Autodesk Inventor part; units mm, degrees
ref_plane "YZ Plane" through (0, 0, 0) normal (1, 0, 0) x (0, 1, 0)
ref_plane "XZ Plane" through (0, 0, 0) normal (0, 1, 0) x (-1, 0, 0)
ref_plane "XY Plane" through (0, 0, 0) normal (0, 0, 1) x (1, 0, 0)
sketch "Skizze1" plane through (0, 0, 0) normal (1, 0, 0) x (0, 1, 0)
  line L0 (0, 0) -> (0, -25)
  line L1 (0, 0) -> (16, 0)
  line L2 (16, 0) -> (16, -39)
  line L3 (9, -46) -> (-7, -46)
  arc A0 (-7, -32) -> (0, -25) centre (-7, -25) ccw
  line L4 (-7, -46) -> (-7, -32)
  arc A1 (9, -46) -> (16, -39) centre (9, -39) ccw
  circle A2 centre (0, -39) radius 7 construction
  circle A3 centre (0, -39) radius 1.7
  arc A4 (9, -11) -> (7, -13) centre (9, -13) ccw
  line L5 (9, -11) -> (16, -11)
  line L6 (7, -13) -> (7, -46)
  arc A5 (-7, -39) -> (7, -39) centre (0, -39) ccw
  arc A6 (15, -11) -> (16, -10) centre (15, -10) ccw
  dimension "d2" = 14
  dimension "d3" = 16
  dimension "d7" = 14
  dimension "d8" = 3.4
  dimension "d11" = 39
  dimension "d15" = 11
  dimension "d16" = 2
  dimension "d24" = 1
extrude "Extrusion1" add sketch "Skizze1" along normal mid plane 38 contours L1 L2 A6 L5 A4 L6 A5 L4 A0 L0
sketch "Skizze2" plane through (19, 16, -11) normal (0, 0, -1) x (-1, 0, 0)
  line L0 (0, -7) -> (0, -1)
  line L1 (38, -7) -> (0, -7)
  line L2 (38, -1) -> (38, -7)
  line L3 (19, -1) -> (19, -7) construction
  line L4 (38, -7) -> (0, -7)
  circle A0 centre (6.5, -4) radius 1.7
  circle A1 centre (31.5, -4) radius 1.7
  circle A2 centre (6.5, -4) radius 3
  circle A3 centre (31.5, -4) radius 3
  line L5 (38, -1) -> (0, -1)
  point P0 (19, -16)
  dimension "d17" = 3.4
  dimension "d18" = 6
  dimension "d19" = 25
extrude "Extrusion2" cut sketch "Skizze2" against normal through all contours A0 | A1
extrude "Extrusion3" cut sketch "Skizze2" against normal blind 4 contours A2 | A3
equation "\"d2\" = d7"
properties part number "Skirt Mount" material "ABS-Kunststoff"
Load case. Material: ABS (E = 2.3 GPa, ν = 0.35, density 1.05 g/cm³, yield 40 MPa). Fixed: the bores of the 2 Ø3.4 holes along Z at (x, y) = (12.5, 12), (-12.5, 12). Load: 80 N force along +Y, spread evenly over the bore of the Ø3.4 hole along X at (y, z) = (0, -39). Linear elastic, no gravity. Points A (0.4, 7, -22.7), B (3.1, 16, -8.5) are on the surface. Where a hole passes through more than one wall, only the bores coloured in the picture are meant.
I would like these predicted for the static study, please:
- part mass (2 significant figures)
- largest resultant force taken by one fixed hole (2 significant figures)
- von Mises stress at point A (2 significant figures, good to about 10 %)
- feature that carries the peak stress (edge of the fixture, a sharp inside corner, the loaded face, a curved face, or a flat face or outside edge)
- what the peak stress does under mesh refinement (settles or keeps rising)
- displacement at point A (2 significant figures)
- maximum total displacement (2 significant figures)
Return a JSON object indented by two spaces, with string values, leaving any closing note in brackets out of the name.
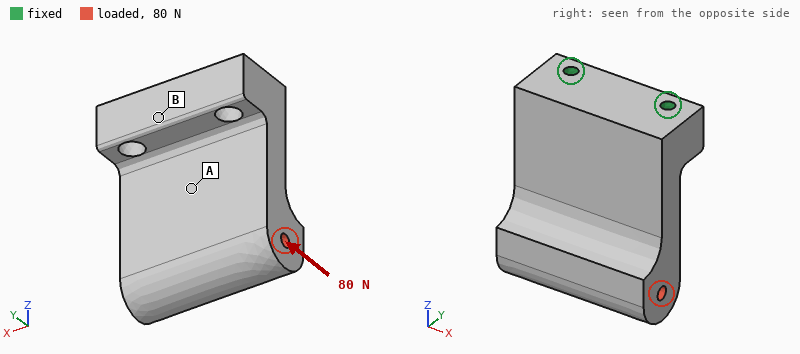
{
  "part mass": "20 g",
  "largest resultant force taken by one fixed hole": "48 N",
  "von Mises stress at point A": "3.9 MPa",
  "feature that carries the peak stress": "edge of the fixture",
  "what the peak stress does under mesh refinement": "keeps rising",
  "displacement at point A": "0.21 mm",
  "maximum total displacement": "0.67 mm"
}
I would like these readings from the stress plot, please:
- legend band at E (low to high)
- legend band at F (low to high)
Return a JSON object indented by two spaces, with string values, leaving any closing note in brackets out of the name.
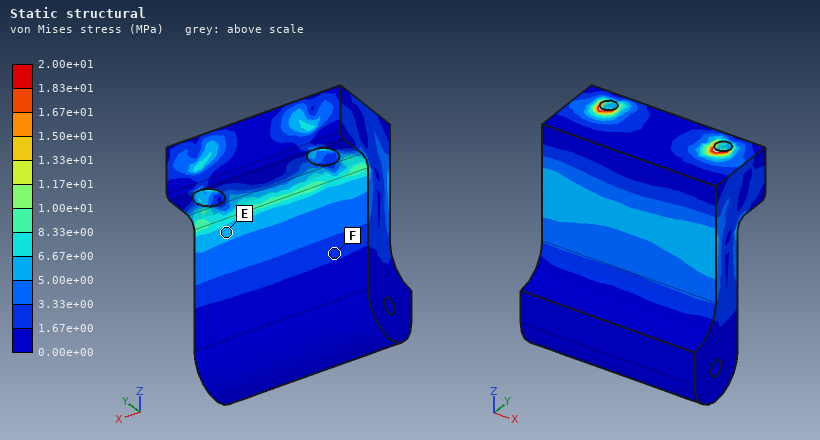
{
  "legend band at E": "5.00e+00 to 6.67e+00 MPa",
  "legend band at F": "1.67e+00 to 3.33e+00 MPa"
}
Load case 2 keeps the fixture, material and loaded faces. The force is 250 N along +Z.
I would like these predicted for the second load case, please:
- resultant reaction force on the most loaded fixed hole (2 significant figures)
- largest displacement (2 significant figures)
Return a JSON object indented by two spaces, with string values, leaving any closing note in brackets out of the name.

{
  "resultant reaction force on the most loaded fixed hole": "130 N",
  "largest displacement": "0.48 mm"
}
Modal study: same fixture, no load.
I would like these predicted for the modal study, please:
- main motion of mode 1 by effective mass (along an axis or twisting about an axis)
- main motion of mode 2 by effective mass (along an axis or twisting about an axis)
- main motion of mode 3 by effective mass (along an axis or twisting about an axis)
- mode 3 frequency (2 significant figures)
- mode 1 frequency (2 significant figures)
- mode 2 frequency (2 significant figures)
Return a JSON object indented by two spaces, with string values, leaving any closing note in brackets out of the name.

{
  "main motion of mode 1 by effective mass": "along Y",
  "main motion of mode 2 by effective mass": "along X",
  "main motion of mode 3 by effective mass": "along X",
  "mode 3 frequency": "2200 Hz",
  "mode 1 frequency": "690 Hz",
  "mode 2 frequency": "2000 Hz"
}
